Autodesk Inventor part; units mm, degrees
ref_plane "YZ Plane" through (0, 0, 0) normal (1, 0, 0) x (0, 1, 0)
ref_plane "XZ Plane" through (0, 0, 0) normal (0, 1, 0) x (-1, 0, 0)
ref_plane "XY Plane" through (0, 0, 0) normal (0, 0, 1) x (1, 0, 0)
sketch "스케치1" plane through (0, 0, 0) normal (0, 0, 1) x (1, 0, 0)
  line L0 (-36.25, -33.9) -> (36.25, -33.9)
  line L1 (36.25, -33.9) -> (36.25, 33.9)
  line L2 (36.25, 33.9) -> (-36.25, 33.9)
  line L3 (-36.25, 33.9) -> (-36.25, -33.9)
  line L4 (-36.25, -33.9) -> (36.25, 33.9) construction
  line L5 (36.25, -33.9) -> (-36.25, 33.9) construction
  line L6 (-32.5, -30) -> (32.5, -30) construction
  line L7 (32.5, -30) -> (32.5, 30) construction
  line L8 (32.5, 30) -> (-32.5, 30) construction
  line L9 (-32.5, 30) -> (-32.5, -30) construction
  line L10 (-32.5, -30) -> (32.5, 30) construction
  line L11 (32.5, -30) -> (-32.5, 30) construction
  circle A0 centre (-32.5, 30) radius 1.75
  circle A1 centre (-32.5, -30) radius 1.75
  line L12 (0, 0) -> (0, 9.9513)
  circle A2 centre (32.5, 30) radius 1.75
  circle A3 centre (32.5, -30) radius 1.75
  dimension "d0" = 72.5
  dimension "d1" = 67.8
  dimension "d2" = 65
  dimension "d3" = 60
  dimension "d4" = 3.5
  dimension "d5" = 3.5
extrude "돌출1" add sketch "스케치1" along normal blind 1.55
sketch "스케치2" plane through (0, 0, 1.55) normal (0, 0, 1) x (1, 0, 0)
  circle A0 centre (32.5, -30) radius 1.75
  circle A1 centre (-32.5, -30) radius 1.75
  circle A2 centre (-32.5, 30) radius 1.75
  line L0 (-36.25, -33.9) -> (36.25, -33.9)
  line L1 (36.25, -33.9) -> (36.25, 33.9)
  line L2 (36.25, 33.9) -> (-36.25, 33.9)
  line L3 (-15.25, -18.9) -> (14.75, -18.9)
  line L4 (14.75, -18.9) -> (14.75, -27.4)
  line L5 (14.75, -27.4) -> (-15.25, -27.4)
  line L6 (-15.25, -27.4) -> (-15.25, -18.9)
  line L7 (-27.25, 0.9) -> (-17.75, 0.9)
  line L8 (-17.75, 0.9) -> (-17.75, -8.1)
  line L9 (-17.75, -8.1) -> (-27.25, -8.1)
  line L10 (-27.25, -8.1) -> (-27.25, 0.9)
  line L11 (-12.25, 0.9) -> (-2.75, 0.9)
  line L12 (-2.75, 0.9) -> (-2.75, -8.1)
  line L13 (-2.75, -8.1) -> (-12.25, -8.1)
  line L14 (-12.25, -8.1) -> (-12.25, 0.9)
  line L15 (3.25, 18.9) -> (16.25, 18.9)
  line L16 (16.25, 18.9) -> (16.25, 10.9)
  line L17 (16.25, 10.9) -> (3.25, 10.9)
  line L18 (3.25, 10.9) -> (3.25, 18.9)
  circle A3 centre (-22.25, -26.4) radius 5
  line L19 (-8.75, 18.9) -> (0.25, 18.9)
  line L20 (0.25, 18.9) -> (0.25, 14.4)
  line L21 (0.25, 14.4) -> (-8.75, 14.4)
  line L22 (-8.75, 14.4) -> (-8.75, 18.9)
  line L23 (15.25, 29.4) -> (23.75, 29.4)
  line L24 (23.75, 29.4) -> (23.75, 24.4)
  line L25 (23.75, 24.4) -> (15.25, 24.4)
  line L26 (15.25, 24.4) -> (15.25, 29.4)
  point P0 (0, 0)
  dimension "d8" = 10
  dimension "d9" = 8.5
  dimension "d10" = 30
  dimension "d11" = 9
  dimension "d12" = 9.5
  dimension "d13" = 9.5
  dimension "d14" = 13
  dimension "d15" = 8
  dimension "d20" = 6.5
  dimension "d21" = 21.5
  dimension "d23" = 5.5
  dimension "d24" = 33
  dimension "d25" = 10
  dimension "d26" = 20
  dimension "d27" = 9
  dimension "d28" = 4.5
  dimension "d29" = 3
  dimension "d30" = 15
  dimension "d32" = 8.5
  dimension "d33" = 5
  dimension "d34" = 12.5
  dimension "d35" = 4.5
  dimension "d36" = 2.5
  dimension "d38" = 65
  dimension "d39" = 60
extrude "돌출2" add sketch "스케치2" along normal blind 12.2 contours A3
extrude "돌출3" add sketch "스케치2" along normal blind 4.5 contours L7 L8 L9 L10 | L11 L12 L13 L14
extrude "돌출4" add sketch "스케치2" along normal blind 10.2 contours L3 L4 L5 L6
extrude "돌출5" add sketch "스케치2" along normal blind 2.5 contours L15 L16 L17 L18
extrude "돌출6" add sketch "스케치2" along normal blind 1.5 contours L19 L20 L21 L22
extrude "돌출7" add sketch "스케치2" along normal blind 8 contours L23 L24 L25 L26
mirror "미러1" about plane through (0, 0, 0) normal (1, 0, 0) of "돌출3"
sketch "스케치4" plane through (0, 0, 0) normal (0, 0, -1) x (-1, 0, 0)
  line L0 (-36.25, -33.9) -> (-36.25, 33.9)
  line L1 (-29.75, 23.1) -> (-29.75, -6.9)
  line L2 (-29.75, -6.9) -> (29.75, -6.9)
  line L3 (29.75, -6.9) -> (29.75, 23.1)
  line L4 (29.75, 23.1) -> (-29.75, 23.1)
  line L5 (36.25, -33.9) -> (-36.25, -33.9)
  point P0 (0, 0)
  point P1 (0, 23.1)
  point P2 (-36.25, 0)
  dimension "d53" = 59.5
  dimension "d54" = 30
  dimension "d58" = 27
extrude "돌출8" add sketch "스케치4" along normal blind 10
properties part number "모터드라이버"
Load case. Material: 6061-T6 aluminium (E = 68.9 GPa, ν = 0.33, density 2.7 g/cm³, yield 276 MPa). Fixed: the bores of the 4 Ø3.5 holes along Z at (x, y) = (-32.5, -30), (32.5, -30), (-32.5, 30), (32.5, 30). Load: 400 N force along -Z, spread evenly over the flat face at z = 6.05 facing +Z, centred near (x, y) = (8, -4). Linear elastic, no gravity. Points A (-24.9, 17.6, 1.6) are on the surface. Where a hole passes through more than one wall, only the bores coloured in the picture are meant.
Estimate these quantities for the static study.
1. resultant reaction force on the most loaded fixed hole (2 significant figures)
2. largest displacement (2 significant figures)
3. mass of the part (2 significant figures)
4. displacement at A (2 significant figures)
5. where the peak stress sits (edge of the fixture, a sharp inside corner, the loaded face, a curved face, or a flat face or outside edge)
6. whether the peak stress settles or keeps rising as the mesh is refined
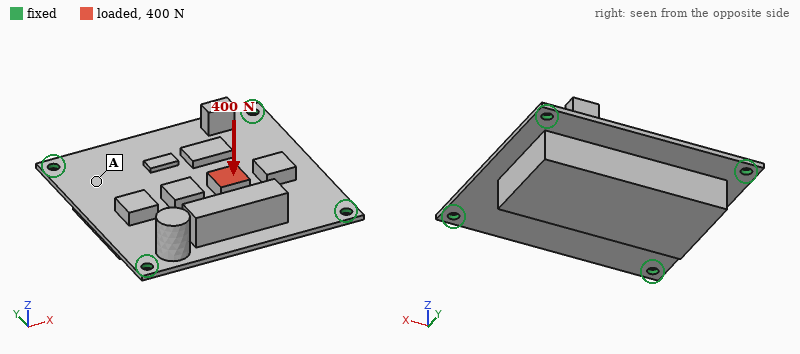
150 N
0.20 mm
84 g
0.050 mm
edge of the fixture
keeps rising
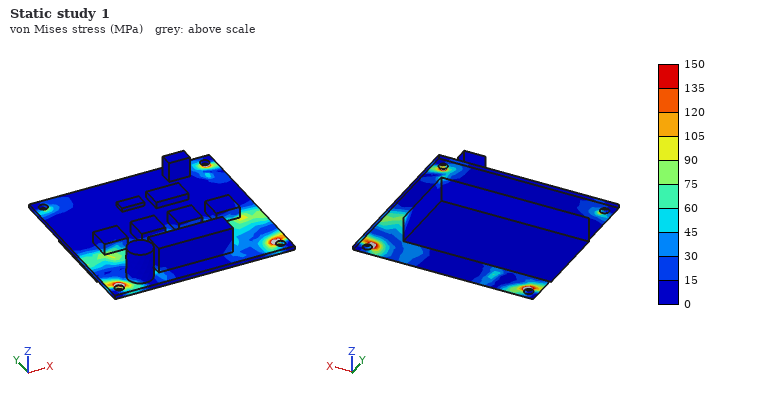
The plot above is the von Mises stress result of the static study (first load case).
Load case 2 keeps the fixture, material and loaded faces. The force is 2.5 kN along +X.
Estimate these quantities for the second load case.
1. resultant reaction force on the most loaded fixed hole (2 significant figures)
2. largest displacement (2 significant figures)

740 N
76 µm
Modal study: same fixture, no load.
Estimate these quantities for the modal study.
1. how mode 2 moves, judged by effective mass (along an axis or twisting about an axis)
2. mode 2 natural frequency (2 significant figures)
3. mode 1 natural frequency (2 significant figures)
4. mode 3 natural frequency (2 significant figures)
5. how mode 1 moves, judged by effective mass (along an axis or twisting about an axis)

twisting about X
2600 Hz
1200 Hz
3100 Hz
along Z
